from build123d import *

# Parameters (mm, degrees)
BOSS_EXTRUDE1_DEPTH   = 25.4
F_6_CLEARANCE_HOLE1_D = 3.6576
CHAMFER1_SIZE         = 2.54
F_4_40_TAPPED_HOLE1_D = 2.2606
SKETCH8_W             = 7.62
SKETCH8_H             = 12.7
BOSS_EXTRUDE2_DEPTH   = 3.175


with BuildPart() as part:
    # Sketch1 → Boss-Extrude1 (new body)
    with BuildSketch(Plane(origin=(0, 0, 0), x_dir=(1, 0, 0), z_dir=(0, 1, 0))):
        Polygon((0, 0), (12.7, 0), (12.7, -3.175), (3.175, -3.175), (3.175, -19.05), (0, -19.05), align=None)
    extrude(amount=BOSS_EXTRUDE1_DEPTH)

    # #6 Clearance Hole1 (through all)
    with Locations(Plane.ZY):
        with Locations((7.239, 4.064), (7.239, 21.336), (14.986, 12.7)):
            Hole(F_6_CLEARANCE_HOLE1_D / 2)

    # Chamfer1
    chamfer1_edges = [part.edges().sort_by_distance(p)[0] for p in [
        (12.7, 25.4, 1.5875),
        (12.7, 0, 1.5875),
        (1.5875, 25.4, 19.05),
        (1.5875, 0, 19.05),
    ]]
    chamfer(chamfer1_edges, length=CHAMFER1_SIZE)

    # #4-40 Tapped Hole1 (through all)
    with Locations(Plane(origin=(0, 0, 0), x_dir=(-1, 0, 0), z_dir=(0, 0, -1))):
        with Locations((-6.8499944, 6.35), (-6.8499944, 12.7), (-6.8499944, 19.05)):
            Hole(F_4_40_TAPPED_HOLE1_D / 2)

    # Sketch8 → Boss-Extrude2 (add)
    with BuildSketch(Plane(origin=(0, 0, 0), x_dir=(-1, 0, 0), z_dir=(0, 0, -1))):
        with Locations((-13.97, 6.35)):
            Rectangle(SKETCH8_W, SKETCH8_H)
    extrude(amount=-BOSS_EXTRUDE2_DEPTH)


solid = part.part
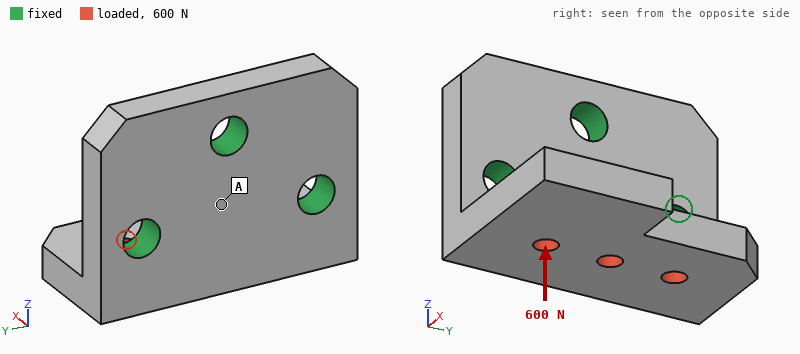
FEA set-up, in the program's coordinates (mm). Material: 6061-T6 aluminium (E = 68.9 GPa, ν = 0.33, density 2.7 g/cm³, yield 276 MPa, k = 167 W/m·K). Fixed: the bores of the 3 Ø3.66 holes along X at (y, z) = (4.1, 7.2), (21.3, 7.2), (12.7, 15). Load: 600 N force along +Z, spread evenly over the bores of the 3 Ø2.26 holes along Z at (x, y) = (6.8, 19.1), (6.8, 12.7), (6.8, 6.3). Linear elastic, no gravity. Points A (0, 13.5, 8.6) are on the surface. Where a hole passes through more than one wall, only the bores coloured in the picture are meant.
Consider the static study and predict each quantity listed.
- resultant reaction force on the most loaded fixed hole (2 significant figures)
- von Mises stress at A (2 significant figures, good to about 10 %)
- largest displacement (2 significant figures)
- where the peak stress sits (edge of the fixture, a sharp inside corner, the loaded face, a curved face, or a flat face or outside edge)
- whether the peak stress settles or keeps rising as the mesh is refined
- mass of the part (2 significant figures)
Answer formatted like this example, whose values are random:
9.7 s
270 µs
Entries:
240 N
14 MPa
72 µm
edge of the fixture
keeps rising
6.3 g
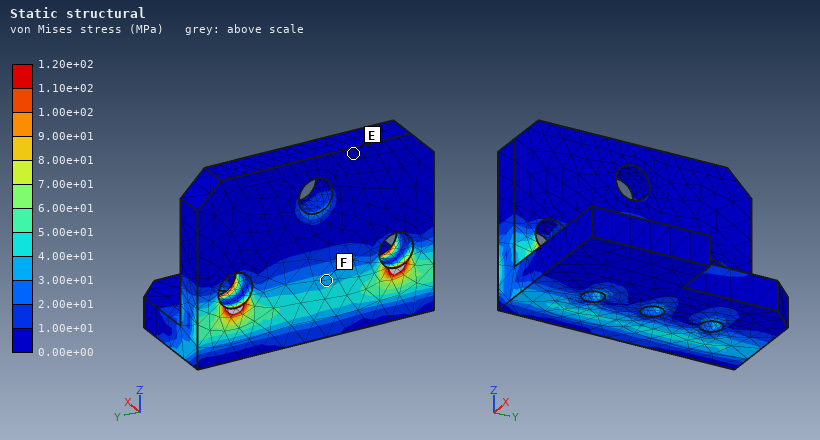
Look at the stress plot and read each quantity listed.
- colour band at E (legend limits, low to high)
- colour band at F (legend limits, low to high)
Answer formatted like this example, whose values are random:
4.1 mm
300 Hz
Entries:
0.00e+00 to 1.00e+01 MPa
3.00e+01 to 4.00e+01 MPa
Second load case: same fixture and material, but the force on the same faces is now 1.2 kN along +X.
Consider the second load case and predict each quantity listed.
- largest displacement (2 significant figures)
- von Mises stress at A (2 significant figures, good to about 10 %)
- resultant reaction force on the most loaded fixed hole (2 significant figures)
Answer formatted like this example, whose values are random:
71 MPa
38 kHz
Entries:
61 µm
31 MPa
650 N
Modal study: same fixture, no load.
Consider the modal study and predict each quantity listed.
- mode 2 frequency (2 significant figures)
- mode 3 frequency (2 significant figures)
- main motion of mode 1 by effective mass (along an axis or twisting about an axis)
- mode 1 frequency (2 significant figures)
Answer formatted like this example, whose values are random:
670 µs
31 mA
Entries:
18 kHz
24 kHz
along Z
8100 Hz
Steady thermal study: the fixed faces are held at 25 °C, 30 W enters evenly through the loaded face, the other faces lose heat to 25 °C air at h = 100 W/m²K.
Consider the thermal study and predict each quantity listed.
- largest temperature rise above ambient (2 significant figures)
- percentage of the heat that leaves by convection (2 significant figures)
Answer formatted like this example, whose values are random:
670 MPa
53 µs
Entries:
25 K
6.0 %
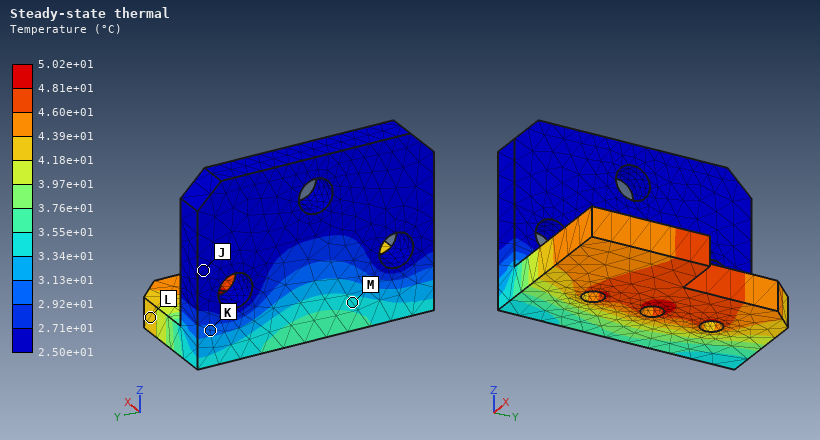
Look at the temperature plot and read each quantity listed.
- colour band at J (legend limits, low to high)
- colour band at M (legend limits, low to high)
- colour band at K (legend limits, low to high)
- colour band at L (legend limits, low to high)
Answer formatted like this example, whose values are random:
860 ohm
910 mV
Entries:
2.50e+01 to 2.71e+01 °C
3.34e+01 to 3.55e+01 °C
2.92e+01 to 3.13e+01 °C
4.18e+01 to 4.39e+01 °C
